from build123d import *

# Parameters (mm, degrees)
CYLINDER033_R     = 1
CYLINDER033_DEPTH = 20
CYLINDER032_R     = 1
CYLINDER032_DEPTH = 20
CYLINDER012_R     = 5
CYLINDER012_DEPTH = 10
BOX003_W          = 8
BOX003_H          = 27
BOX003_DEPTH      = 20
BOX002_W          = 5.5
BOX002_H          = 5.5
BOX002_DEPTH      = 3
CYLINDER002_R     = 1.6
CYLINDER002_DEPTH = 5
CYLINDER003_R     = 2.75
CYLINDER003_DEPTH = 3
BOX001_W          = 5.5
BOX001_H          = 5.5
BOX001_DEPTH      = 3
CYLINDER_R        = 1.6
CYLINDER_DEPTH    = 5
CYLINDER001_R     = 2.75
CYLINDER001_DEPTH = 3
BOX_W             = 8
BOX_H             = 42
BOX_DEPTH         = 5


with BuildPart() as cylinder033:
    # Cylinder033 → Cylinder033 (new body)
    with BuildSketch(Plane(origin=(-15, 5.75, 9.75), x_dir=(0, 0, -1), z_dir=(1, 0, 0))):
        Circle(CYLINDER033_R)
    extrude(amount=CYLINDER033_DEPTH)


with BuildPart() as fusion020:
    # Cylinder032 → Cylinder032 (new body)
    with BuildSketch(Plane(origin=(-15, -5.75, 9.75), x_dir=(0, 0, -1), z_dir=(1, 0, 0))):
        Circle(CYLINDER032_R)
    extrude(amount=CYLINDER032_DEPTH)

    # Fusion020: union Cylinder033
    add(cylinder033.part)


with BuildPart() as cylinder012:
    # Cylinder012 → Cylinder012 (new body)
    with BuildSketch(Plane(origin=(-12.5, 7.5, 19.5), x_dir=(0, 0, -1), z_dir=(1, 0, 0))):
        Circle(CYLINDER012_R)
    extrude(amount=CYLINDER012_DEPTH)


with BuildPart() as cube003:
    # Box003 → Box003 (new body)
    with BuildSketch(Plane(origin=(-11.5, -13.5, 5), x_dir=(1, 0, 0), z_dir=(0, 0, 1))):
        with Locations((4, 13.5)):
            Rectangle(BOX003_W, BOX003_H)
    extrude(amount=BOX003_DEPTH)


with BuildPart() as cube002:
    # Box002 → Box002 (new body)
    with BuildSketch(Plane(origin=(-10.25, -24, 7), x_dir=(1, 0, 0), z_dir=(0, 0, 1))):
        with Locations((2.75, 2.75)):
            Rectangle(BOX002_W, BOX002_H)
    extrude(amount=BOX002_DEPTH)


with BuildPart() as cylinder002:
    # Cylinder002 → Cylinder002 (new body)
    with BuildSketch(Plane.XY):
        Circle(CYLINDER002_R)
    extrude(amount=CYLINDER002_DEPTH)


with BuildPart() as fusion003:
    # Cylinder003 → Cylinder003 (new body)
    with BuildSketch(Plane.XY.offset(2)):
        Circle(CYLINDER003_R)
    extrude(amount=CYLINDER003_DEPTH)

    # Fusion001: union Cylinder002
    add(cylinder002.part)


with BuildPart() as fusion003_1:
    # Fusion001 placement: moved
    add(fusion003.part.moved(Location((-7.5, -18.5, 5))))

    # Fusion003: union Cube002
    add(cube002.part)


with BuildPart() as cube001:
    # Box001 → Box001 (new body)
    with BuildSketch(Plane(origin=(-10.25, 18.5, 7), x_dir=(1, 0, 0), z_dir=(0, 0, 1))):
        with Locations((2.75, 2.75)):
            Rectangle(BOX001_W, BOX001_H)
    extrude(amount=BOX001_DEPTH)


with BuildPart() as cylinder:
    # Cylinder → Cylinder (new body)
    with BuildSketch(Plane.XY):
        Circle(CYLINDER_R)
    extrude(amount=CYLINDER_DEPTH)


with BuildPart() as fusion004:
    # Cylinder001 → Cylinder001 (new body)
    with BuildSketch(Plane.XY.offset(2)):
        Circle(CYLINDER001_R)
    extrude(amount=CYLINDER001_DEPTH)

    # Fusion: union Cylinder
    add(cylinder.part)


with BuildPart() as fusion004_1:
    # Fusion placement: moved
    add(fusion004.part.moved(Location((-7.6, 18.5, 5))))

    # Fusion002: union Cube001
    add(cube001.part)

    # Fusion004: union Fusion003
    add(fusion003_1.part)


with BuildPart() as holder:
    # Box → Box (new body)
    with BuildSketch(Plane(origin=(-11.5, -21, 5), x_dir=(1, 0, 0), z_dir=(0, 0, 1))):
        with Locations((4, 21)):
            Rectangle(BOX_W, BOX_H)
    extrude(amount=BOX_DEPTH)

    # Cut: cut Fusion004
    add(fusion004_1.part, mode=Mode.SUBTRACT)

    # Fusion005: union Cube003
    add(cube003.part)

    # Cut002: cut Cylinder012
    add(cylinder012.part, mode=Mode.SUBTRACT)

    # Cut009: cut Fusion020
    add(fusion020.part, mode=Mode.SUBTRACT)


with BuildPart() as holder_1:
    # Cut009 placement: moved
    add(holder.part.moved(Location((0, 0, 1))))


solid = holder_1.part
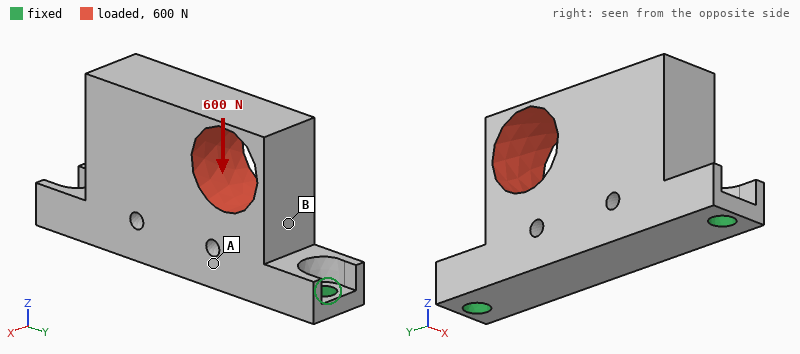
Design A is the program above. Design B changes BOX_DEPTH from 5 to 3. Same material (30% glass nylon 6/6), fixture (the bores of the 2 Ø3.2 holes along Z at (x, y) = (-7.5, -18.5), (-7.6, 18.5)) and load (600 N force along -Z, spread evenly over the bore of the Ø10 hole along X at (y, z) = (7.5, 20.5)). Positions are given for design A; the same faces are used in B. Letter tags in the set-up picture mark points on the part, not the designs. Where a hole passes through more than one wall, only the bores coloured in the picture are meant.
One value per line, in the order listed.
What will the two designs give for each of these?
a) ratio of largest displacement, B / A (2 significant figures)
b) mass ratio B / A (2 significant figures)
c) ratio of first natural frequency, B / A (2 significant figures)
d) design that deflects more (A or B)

1.3
0.97
0.77
B
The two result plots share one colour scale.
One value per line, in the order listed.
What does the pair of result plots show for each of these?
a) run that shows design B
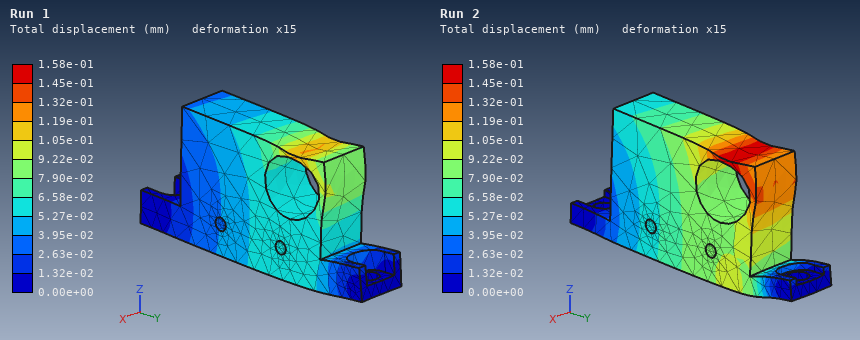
Run 2
